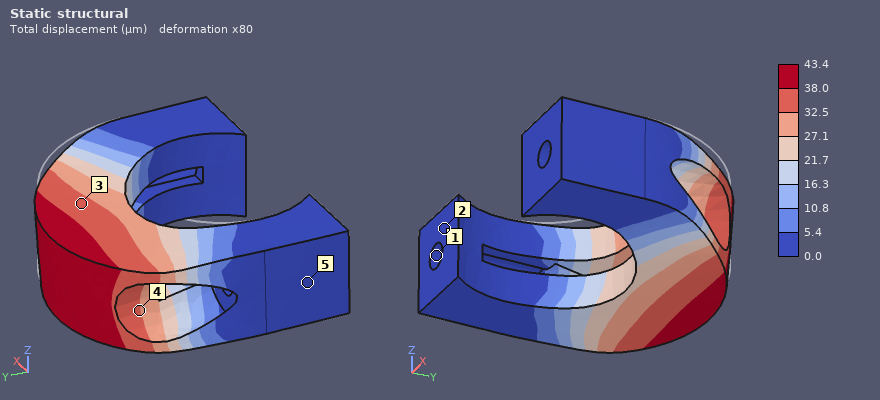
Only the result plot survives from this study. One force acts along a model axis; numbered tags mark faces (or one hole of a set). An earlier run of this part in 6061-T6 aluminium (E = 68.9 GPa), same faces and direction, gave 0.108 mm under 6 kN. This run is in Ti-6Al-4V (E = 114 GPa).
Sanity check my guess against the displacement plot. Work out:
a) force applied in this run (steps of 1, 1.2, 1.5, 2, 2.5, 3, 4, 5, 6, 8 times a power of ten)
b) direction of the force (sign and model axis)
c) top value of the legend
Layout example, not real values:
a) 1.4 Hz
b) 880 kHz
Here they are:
a) 4 kN
b) -Z
c) 43.4 µm
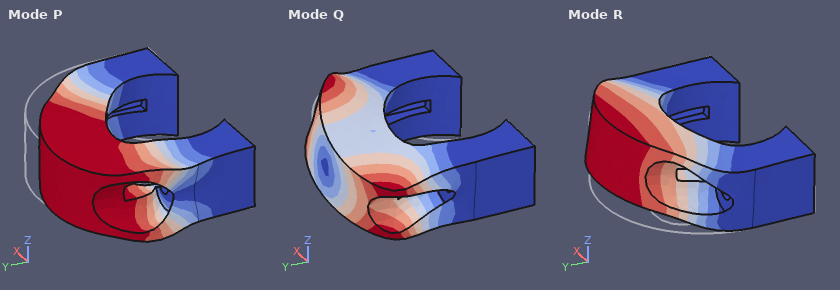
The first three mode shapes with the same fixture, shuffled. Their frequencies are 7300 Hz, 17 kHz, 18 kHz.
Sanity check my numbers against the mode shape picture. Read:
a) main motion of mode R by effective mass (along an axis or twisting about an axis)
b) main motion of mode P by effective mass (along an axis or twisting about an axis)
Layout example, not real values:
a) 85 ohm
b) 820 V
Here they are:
a) along Z
b) along X
